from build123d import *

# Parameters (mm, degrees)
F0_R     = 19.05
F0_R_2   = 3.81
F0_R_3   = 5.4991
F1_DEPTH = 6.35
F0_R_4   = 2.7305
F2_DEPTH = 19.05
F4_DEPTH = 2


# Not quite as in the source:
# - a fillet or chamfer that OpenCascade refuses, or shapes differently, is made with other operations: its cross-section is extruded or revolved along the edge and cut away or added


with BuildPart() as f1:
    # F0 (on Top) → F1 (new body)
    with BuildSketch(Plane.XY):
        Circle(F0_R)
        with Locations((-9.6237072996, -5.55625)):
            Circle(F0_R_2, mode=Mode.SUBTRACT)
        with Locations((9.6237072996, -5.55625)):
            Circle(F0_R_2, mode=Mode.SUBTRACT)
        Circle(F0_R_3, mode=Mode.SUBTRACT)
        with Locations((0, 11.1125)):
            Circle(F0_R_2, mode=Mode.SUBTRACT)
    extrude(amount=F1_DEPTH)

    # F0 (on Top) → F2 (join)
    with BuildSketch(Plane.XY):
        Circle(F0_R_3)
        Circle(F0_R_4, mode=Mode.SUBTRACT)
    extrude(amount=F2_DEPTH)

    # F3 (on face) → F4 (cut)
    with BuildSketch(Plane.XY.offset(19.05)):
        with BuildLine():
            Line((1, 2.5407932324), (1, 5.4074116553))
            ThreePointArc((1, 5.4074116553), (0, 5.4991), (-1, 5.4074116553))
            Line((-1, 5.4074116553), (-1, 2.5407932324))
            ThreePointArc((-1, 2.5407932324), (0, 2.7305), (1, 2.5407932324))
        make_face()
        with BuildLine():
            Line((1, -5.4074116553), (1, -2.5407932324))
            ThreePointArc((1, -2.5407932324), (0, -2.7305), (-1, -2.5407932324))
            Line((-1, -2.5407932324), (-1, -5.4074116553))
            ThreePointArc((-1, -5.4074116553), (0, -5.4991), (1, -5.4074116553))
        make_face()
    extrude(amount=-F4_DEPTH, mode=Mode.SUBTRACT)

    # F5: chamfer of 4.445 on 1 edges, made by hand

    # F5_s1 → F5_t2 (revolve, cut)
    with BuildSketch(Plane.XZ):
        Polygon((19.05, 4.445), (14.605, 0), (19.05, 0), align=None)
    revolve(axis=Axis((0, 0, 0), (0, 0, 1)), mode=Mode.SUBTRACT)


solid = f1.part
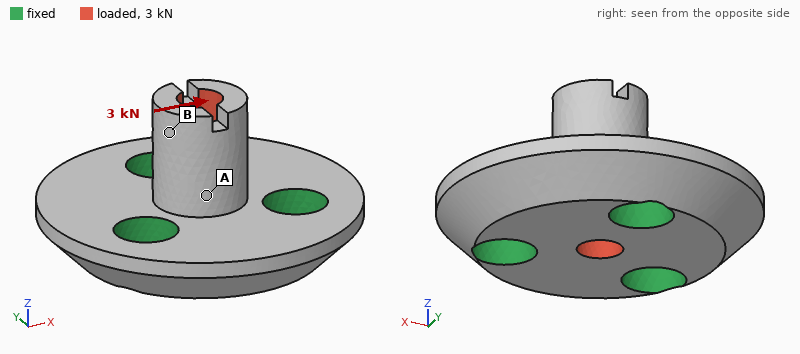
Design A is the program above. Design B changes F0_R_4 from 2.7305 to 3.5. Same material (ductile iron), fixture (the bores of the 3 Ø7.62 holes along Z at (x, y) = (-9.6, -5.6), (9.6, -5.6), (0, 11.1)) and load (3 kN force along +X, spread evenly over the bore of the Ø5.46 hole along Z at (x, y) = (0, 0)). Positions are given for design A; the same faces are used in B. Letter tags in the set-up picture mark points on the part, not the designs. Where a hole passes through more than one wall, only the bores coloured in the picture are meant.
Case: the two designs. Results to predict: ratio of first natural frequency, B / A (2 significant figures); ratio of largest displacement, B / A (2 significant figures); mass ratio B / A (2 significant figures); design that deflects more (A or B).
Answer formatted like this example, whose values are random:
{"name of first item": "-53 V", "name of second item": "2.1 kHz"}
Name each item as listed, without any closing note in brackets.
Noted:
{"ratio of first natural frequency, B / A": "1.0", "ratio of largest displacement, B / A": "1.2", "mass ratio B / A": "0.95", "design that deflects more": "B"}
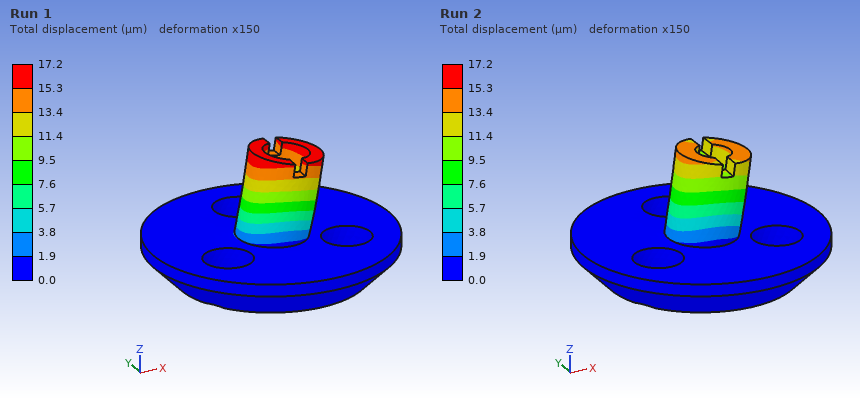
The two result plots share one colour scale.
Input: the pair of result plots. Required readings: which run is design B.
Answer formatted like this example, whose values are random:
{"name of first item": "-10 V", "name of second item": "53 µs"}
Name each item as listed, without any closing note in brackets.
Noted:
{"which run is design B": "Run 1"}
